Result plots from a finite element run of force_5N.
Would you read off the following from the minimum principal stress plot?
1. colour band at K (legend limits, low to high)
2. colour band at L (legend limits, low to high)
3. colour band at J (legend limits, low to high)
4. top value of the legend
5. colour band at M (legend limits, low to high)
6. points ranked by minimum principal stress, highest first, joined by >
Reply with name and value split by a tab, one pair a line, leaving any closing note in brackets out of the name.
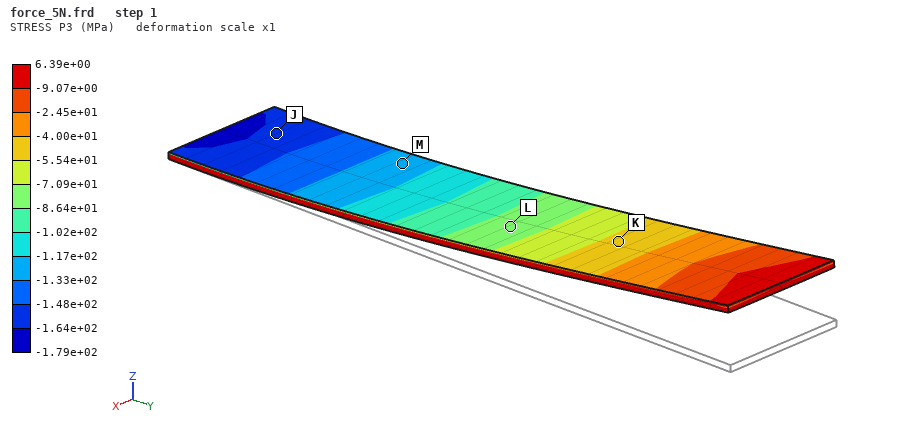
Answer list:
colour band at K	-5.54e+01 to -4.00e+01 MPa
colour band at L	-8.64e+01 to -7.09e+01 MPa
colour band at J	-1.64e+02 to -1.48e+02 MPa
top value of the legend	6.39e+00 MPa
colour band at M	-1.33e+02 to -1.17e+02 MPa
points ranked by minimum principal stress, highest first, joined by >	K > L > M > J
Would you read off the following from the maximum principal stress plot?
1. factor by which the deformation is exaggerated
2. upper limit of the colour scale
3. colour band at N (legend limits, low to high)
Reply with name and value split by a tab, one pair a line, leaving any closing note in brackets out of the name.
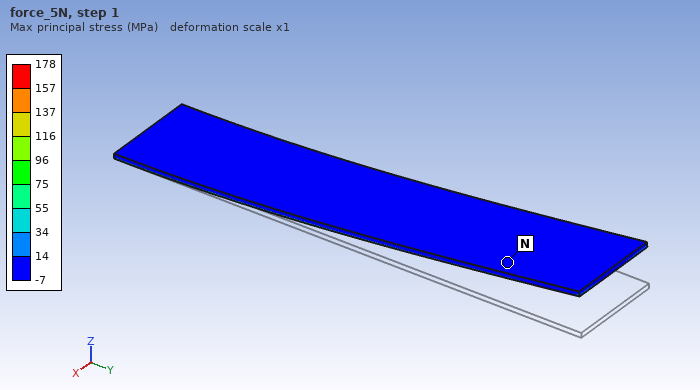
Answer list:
factor by which the deformation is exaggerated	1
upper limit of the colour scale	178 MPa
colour band at N	-7 to 14 MPa
